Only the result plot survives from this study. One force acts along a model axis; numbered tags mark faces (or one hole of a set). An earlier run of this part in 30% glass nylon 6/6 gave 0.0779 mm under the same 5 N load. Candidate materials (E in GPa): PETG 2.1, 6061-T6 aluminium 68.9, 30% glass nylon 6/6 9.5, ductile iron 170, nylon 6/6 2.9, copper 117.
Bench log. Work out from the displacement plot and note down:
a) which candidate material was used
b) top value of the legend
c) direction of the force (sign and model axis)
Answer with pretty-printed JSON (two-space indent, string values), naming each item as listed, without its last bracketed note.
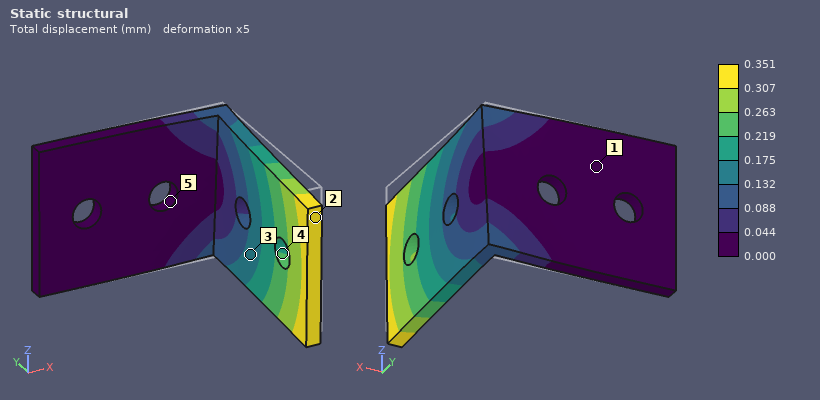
{
  "which candidate material was used": "PETG",
  "top value of the legend": "0.351 mm",
  "direction of the force": "-Z"
}
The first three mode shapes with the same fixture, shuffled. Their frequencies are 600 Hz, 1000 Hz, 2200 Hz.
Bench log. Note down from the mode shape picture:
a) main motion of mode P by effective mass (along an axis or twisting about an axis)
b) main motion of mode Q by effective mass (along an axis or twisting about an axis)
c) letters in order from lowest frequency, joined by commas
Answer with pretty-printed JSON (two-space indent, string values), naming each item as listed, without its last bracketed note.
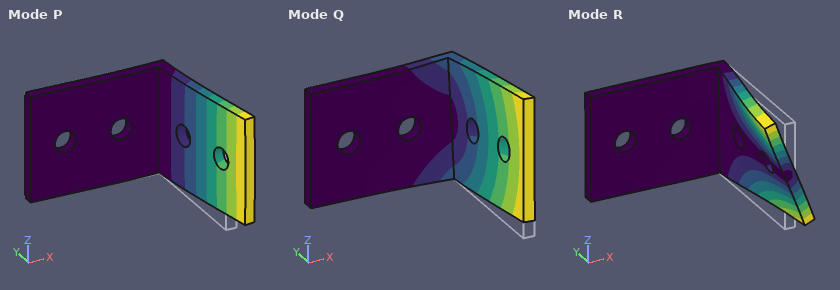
{
  "main motion of mode P by effective mass": "along X",
  "main motion of mode Q by effective mass": "along Z",
  "letters in order from lowest frequency, joined by commas": "P, Q, R"
}
